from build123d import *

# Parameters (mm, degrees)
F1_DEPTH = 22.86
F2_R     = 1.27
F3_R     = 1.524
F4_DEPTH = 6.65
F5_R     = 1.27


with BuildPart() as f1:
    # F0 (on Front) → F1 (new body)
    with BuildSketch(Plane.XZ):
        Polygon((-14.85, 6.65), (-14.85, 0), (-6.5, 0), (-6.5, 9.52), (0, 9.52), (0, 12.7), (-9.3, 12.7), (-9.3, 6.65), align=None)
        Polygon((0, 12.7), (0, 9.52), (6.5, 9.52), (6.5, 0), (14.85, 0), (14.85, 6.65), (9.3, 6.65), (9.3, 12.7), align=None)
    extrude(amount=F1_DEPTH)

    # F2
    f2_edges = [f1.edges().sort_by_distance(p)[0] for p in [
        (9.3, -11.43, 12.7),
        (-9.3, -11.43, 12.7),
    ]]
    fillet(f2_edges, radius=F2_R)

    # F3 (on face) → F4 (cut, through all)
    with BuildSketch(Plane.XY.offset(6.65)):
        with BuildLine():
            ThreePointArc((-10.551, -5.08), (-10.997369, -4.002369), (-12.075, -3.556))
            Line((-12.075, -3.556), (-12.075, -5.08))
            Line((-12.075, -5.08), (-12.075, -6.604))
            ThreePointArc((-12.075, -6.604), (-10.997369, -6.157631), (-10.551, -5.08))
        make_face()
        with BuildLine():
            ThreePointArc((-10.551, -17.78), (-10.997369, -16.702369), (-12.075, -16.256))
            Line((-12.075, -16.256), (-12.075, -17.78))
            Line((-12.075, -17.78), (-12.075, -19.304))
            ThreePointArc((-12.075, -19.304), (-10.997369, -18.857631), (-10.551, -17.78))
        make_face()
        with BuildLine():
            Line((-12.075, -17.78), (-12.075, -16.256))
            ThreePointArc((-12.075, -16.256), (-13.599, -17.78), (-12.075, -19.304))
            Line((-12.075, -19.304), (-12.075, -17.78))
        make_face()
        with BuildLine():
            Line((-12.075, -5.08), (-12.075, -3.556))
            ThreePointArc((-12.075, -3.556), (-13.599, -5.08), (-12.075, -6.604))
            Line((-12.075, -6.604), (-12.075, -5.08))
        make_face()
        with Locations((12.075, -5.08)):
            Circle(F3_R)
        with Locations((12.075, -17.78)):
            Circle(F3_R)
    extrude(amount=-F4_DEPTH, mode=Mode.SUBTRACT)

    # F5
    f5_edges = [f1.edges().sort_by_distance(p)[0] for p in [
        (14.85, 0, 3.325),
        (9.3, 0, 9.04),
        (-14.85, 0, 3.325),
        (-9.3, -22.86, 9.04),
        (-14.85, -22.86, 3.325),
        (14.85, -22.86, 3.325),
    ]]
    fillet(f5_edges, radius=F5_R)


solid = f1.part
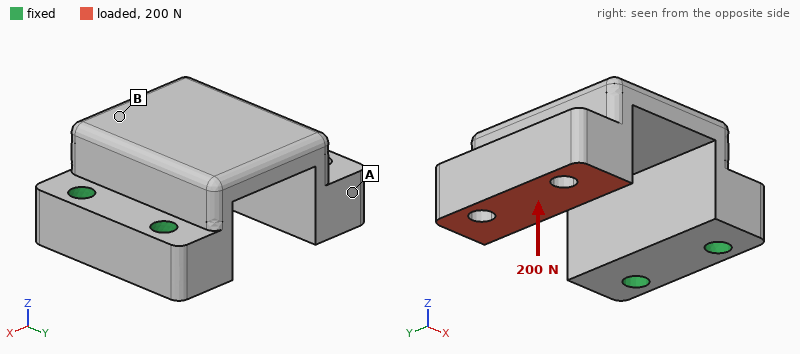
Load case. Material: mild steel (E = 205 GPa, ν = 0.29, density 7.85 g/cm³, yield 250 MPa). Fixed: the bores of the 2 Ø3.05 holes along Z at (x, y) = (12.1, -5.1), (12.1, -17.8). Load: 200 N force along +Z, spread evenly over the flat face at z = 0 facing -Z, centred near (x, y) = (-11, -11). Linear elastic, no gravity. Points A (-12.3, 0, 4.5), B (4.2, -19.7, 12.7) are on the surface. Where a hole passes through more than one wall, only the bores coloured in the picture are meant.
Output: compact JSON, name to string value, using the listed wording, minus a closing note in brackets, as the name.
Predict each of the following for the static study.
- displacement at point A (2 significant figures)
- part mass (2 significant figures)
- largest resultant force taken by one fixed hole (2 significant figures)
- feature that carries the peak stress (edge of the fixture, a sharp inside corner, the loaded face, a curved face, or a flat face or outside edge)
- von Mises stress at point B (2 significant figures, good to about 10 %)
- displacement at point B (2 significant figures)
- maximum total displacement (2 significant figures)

{"displacement at point A": "0.088 mm", "part mass": "32 g", "largest resultant force taken by one fixed hole": "100 N", "feature that carries the peak stress": "a sharp inside corner", "von Mises stress at point B": "75 MPa", "displacement at point B": "0.017 mm", "maximum total displacement": "0.11 mm"}
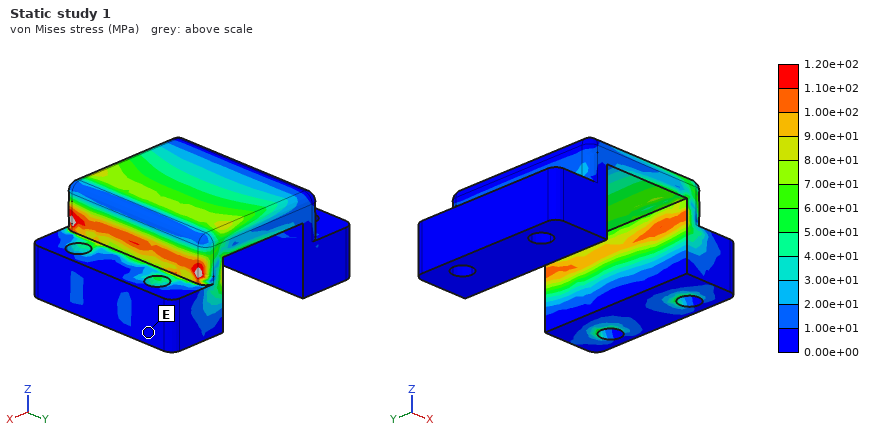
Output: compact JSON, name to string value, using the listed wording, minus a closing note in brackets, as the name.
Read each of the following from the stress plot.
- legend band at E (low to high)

{"legend band at E": "0.00e+00 to 1.00e+01 MPa"}
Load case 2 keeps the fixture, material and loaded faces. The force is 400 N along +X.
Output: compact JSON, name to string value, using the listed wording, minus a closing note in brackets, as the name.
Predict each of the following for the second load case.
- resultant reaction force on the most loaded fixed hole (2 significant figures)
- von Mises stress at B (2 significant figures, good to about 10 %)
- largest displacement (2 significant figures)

{"resultant reaction force on the most loaded fixed hole": "200 N", "von Mises stress at B": "110 MPa", "largest displacement": "0.16 mm"}
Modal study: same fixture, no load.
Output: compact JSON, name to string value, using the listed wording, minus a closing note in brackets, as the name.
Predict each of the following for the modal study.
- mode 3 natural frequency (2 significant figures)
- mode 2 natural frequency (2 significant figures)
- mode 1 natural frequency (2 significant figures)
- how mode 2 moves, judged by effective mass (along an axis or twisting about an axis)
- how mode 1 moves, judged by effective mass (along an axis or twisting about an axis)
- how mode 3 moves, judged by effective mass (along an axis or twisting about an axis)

{"mode 3 natural frequency": "7400 Hz", "mode 2 natural frequency": "4300 Hz", "mode 1 natural frequency": "2200 Hz", "how mode 2 moves, judged by effective mass": "along Y", "how mode 1 moves, judged by effective mass": "along Z", "how mode 3 moves, judged by effective mass": "along X"}
